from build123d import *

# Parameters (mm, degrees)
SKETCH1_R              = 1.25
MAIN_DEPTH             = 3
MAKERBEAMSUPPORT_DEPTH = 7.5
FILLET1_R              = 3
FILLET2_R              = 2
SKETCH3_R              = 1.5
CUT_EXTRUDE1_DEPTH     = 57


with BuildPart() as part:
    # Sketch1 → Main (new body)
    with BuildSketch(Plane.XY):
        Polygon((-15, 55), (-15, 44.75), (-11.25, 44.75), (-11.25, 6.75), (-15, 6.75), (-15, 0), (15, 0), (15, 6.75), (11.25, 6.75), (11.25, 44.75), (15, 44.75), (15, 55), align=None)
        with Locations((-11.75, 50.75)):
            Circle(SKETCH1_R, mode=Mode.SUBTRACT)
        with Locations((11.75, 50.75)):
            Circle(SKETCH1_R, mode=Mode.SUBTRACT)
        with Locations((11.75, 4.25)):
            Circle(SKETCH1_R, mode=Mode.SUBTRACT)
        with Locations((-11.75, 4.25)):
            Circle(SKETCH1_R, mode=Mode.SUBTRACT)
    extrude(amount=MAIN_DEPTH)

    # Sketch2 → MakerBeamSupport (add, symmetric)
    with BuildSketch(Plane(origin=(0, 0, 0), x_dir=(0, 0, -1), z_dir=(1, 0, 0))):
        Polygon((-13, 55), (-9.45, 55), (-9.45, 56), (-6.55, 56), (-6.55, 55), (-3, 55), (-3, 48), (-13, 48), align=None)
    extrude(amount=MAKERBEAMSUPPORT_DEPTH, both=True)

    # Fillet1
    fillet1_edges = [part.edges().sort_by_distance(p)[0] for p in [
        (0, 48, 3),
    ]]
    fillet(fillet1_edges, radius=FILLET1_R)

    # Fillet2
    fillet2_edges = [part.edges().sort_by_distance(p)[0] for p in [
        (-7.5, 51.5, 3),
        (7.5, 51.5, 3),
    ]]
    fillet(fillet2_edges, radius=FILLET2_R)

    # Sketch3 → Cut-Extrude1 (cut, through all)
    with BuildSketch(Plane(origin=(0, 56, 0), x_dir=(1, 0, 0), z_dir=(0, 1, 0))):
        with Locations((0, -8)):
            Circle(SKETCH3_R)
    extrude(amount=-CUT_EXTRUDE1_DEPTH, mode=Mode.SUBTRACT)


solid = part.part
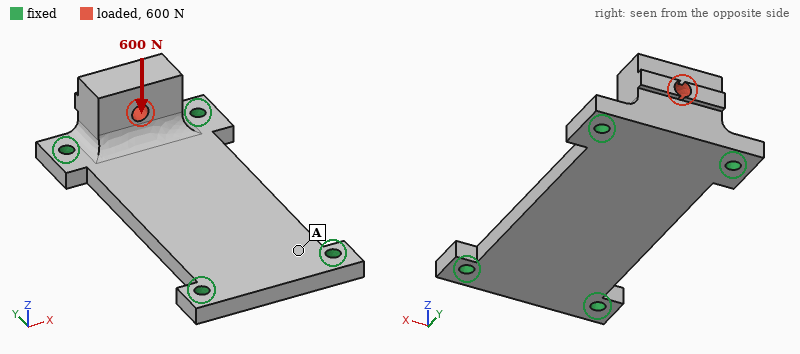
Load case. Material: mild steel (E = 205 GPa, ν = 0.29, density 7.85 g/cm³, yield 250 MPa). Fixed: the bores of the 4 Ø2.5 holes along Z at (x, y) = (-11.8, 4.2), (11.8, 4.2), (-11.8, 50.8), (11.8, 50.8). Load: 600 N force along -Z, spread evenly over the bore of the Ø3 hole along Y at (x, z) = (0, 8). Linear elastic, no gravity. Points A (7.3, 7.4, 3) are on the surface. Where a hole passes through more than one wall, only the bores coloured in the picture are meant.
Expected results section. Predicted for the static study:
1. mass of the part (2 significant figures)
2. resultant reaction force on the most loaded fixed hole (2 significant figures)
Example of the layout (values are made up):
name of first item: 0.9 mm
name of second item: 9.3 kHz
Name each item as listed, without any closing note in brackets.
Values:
mass of the part: 40 g
resultant reaction force on the most loaded fixed hole: 350 N
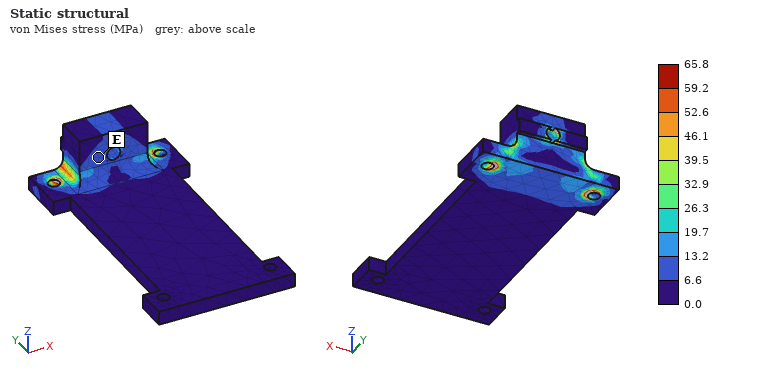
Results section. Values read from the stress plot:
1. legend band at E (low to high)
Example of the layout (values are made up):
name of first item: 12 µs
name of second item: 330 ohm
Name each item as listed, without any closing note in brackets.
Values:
legend band at E: 6.6 to 13.2 MPa
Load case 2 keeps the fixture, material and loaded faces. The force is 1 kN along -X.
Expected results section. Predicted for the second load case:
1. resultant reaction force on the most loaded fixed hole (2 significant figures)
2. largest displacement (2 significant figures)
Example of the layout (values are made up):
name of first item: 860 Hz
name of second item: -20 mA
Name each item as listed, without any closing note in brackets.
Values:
resultant reaction force on the most loaded fixed hole: 600 N
largest displacement: 3.3 µm
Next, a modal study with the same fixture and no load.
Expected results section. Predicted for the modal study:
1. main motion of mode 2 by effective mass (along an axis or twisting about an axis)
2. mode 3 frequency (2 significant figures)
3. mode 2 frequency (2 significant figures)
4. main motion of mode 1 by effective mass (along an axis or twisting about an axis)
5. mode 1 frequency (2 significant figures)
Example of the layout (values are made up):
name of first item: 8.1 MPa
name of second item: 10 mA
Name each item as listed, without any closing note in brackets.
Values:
main motion of mode 2 by effective mass: twisting about Y
mode 3 frequency: 14 kHz
mode 2 frequency: 12 kHz
main motion of mode 1 by effective mass: along Z
mode 1 frequency: 6300 Hz
